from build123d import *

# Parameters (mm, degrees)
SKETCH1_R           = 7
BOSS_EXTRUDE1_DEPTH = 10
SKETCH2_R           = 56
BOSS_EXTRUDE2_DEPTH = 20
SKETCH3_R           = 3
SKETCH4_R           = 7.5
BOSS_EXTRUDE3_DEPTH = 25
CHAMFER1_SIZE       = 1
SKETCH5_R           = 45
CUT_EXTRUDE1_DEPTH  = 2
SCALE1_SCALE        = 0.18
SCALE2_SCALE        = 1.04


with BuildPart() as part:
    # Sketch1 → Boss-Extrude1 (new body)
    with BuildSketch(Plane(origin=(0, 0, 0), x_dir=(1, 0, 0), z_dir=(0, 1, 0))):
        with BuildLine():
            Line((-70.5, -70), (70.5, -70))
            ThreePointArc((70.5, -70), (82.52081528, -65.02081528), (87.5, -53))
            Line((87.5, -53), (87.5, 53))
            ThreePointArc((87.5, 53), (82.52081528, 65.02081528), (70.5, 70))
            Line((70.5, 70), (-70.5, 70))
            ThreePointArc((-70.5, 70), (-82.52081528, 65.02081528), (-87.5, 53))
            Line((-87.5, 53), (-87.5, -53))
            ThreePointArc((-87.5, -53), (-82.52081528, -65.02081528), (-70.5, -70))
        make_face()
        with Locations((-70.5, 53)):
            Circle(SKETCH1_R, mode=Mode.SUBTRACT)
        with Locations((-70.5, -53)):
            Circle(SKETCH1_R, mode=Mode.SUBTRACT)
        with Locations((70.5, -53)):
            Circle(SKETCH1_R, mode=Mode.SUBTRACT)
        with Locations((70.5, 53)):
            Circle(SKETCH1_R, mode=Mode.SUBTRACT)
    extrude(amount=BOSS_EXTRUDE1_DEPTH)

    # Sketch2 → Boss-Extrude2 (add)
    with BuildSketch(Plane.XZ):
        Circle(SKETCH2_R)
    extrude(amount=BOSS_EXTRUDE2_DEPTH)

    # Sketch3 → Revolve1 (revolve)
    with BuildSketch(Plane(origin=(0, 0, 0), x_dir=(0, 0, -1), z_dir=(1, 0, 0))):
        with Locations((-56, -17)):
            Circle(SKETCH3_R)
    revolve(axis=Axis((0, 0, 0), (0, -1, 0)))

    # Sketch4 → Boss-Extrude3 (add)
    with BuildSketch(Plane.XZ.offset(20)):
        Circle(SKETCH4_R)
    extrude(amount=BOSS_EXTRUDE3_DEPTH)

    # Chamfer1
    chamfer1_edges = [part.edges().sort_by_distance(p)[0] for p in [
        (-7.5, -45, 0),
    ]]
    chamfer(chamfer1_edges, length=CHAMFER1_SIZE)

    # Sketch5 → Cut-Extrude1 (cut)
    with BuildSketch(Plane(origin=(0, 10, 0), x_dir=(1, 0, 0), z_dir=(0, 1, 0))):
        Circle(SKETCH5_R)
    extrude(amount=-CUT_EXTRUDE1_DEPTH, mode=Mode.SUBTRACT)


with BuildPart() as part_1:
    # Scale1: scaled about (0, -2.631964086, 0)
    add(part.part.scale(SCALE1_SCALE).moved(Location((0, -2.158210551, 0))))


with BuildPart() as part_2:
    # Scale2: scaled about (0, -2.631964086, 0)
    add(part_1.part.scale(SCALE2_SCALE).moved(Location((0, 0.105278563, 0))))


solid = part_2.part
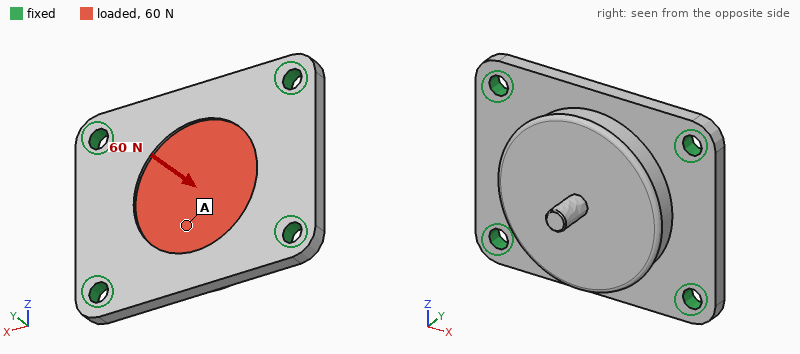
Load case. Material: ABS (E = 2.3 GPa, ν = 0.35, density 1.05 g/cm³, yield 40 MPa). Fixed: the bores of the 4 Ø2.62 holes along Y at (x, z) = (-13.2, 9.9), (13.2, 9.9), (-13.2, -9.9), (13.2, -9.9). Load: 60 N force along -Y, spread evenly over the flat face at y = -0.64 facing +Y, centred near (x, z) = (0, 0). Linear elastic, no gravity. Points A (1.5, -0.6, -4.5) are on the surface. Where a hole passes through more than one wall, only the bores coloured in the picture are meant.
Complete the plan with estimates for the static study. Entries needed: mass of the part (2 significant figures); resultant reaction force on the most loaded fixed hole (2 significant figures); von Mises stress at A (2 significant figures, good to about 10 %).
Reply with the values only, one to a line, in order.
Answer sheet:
3.0 g
18 N
1.0 MPa
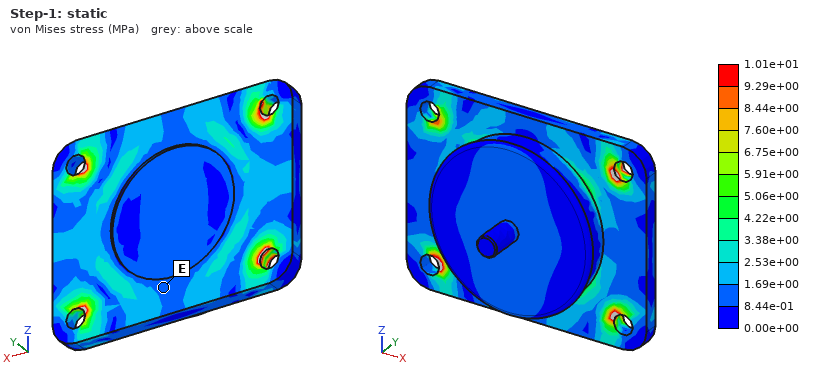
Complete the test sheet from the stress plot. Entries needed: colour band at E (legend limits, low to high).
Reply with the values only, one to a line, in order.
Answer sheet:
8.44e-01 to 1.69e+00 MPa
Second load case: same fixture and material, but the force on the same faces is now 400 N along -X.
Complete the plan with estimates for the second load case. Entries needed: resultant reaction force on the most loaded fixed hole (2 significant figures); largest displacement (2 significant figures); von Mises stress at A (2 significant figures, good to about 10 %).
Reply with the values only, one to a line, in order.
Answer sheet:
100 N
40 µm
4.2 MPa
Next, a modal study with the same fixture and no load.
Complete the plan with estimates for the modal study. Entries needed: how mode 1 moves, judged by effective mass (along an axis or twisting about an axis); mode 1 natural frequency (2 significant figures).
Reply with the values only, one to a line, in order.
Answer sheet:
along Y
4000 Hz
